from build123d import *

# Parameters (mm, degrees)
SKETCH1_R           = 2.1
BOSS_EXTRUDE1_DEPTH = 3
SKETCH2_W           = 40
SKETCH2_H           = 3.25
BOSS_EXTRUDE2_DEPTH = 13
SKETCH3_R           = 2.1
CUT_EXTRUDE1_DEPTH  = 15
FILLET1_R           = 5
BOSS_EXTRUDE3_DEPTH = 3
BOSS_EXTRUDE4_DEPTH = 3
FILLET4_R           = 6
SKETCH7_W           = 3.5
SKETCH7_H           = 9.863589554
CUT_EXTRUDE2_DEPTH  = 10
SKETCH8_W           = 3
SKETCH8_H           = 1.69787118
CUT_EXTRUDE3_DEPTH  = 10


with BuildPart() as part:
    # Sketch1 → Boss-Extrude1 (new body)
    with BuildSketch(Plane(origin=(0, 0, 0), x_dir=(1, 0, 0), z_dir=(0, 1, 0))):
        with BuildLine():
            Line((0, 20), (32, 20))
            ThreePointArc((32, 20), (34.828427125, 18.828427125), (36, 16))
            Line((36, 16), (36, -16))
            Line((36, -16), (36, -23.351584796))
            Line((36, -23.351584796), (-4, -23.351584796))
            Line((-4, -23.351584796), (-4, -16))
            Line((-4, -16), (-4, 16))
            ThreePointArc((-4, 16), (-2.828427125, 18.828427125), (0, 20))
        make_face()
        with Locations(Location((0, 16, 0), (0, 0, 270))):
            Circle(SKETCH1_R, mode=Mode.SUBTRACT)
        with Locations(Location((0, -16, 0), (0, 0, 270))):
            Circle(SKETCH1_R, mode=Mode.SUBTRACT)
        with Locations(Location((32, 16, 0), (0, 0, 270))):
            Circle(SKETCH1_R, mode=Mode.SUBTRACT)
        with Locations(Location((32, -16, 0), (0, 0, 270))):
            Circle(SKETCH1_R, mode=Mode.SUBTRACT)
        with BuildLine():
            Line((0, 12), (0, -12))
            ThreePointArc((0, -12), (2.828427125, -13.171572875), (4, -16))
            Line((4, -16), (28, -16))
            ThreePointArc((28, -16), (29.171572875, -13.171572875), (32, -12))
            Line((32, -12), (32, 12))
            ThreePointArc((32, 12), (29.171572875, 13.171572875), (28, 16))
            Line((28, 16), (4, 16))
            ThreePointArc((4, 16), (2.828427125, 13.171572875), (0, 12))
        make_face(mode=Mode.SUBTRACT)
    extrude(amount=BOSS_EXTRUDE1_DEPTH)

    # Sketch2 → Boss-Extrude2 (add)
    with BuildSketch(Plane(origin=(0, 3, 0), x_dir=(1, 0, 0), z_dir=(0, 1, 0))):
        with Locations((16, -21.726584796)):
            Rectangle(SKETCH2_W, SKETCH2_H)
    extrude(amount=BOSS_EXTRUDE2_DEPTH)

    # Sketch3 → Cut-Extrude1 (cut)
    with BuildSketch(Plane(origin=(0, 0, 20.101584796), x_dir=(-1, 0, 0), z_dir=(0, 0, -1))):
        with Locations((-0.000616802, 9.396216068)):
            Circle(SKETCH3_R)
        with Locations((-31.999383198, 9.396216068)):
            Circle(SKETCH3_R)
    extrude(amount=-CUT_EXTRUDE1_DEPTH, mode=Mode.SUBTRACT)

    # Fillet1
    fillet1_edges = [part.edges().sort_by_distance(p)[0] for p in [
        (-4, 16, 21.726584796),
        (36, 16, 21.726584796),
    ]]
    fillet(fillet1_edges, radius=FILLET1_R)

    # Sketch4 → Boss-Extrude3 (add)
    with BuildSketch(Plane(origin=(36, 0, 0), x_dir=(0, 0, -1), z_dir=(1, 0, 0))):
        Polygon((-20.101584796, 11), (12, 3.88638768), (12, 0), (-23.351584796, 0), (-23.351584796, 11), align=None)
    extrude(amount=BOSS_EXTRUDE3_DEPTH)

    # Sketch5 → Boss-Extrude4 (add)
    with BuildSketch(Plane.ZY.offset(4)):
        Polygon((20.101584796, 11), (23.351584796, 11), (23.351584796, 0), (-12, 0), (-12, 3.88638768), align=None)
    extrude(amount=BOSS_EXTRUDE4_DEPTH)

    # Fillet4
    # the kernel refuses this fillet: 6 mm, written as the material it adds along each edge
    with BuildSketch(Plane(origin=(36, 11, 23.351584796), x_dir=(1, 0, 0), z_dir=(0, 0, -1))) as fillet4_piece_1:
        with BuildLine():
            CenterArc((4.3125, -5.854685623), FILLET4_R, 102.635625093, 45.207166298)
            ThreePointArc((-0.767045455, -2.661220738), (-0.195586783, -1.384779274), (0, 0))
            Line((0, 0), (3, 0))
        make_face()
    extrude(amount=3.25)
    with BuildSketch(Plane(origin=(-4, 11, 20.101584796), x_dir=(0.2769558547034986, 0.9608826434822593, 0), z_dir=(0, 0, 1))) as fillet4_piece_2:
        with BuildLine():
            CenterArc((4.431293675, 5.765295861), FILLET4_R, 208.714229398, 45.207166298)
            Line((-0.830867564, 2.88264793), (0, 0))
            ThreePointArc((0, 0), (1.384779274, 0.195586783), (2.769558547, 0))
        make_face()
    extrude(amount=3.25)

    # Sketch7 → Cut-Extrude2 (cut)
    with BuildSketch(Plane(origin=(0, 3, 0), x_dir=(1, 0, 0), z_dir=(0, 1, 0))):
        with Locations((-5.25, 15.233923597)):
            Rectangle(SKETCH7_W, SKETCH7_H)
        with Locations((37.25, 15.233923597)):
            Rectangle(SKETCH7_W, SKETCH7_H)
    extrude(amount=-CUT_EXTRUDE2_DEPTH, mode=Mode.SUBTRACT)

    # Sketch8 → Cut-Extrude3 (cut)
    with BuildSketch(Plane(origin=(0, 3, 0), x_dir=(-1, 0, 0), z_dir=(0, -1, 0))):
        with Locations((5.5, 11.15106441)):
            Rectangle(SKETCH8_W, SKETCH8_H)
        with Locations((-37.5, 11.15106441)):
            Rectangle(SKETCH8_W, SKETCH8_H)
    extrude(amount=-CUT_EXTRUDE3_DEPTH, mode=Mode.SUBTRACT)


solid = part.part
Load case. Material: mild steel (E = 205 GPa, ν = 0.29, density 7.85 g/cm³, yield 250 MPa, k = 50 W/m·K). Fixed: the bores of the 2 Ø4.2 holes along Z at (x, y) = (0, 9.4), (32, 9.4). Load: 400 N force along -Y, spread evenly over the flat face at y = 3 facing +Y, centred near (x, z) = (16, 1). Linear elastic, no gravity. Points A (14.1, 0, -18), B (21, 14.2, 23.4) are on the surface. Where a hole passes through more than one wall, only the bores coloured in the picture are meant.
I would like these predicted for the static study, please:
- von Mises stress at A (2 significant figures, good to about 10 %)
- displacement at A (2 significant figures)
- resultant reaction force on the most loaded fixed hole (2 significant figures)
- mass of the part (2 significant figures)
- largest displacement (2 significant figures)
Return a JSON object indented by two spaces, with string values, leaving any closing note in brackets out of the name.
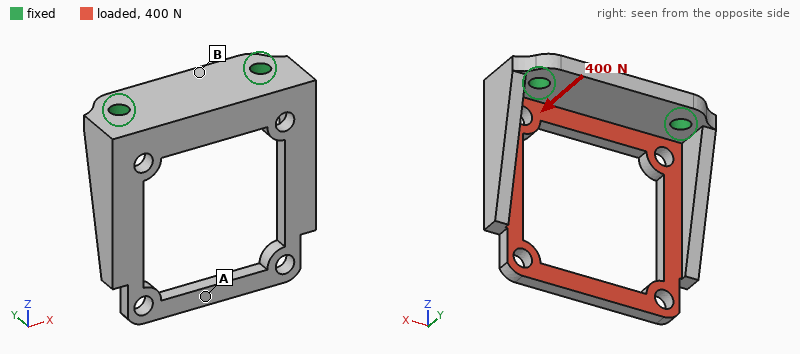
{
  "von Mises stress at A": "65 MPa",
  "displacement at A": "0.14 mm",
  "resultant reaction force on the most loaded fixed hole": "210 N",
  "mass of the part": "41 g",
  "largest displacement": "0.15 mm"
}
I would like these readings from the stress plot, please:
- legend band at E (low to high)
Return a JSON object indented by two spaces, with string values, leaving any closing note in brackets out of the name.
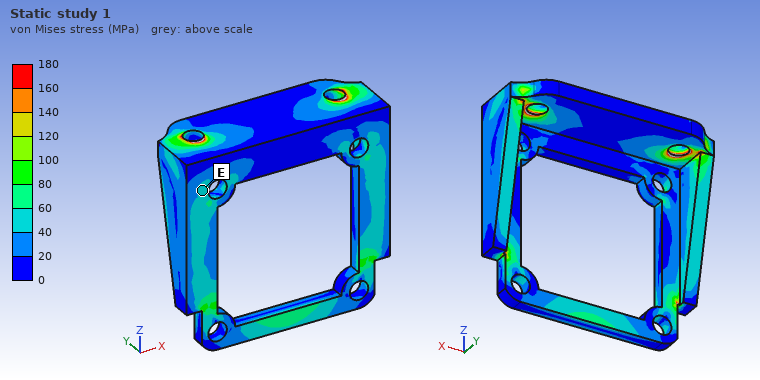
{
  "legend band at E": "40 to 60 MPa"
}
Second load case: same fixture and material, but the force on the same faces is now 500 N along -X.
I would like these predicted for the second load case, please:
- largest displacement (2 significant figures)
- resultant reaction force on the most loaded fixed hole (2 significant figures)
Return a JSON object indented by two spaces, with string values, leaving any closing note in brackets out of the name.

{
  "largest displacement": "74 µm",
  "resultant reaction force on the most loaded fixed hole": "360 N"
}
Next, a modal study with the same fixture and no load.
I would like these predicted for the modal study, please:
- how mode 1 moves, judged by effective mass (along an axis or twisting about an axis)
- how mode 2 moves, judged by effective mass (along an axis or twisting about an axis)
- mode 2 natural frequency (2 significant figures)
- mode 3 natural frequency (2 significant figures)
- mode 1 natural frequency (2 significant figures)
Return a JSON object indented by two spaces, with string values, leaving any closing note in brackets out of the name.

{
  "how mode 1 moves, judged by effective mass": "along Y",
  "how mode 2 moves, judged by effective mass": "along X",
  "mode 2 natural frequency": "3200 Hz",
  "mode 3 natural frequency": "5000 Hz",
  "mode 1 natural frequency": "2600 Hz"
}
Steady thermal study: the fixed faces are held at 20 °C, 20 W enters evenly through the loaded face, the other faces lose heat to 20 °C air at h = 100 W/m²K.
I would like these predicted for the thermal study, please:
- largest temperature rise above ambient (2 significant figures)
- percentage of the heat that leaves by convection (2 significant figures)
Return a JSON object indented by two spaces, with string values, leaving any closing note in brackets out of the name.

{
  "largest temperature rise above ambient": "83 K",
  "percentage of the heat that leaves by convection": "50 %"
}
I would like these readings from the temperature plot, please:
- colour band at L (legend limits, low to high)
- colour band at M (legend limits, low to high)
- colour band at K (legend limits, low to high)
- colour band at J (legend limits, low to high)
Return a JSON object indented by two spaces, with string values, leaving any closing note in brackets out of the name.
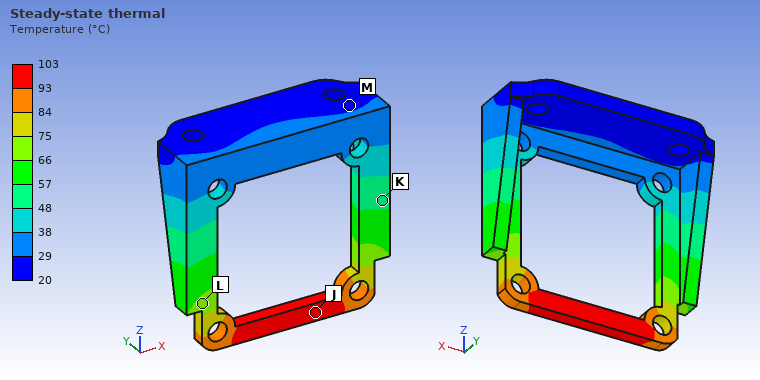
{
  "colour band at L": "66 to 75 °C",
  "colour band at M": "20 to 29 °C",
  "colour band at K": "48 to 57 °C",
  "colour band at J": "93 to 103 °C"
}
